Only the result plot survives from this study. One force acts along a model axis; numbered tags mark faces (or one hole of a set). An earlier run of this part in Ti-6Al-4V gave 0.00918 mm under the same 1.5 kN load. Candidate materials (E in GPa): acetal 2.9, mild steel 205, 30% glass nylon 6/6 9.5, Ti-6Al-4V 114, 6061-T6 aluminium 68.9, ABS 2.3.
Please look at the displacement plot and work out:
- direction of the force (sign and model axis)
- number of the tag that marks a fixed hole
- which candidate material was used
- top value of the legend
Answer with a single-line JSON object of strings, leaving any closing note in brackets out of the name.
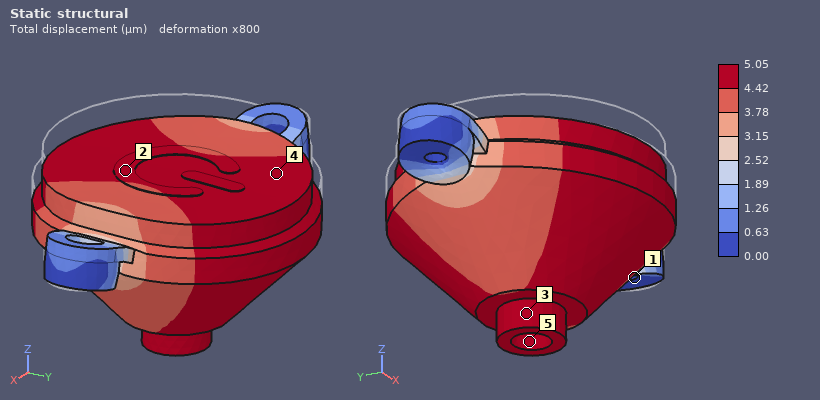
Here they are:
{"direction of the force": "-Z", "number of the tag that marks a fixed hole": "1", "which candidate material was used": "mild steel", "top value of the legend": "5.05 µm"}
